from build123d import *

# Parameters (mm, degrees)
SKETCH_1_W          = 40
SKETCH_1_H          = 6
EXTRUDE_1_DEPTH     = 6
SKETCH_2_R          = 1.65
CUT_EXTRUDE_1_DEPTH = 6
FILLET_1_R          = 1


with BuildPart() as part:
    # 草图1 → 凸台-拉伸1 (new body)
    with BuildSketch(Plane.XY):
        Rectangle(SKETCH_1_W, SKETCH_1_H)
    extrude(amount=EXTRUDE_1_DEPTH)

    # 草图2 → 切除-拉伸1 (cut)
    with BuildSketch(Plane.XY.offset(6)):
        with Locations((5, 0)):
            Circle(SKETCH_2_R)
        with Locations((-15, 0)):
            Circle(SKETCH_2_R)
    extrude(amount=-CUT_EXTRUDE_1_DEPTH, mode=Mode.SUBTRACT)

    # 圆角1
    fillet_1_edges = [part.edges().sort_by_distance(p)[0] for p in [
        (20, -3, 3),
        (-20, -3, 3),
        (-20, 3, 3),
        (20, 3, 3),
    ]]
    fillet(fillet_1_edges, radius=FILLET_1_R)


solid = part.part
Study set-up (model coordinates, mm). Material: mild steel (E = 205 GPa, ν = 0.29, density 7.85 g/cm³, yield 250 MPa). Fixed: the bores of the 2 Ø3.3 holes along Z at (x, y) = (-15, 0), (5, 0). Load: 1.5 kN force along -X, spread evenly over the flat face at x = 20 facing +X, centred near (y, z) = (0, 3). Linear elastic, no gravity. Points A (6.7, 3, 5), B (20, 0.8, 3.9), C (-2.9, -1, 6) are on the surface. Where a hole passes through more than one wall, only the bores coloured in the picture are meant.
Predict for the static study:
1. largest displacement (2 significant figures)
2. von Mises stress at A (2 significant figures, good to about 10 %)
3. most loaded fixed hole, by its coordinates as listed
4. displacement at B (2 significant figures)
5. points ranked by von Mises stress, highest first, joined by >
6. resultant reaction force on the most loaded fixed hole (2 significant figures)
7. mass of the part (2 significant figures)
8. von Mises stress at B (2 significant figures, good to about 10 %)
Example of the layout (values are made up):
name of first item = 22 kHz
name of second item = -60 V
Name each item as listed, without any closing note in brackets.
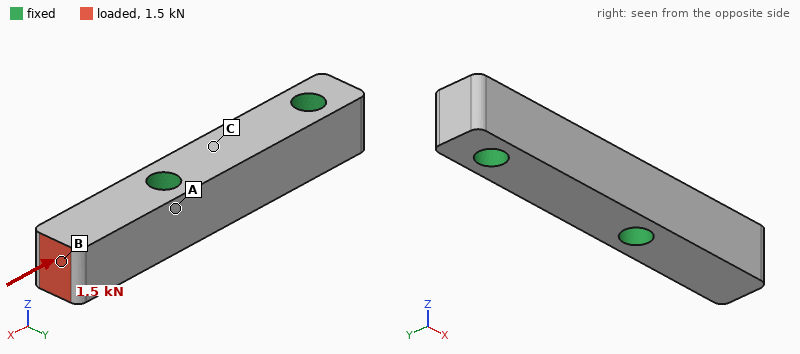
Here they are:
largest displacement = 3.2 µm
von Mises stress at A = 24 MPa
most loaded fixed hole, by its coordinates as listed = (5, 0)
displacement at B = 3.1 µm
points ranked by von Mises stress, highest first, joined by > = B > A > C
resultant reaction force on the most loaded fixed hole = 1.5 kN
mass of the part = 10 g
von Mises stress at B = 47 MPa
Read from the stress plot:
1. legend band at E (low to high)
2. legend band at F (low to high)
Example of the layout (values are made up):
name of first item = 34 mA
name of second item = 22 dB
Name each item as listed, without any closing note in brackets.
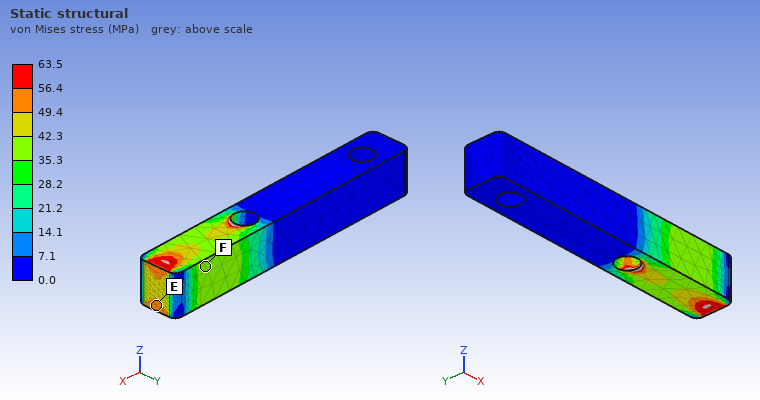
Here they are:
legend band at E = 49.4 to 56.4 MPa
legend band at F = 35.3 to 42.3 MPa
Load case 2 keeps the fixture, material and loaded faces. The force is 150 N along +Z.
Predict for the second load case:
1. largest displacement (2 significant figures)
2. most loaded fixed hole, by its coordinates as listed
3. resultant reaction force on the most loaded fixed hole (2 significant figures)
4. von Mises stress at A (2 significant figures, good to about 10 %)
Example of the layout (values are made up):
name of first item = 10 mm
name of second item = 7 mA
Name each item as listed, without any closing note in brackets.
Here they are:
largest displacement = 7.5 µm
most loaded fixed hole, by its coordinates as listed = (5, 0)
resultant reaction force on the most loaded fixed hole = 150 N
von Mises stress at A = 20 MPa
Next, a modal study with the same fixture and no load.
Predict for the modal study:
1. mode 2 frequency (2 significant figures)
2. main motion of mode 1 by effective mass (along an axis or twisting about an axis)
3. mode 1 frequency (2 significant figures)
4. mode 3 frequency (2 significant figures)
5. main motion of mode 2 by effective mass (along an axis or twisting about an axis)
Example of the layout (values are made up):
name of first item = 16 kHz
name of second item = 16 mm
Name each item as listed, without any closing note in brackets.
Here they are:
mode 2 frequency = 23 kHz
main motion of mode 1 by effective mass = along Y
mode 1 frequency = 20 kHz
mode 3 frequency = 53 kHz
main motion of mode 2 by effective mass = along Z
